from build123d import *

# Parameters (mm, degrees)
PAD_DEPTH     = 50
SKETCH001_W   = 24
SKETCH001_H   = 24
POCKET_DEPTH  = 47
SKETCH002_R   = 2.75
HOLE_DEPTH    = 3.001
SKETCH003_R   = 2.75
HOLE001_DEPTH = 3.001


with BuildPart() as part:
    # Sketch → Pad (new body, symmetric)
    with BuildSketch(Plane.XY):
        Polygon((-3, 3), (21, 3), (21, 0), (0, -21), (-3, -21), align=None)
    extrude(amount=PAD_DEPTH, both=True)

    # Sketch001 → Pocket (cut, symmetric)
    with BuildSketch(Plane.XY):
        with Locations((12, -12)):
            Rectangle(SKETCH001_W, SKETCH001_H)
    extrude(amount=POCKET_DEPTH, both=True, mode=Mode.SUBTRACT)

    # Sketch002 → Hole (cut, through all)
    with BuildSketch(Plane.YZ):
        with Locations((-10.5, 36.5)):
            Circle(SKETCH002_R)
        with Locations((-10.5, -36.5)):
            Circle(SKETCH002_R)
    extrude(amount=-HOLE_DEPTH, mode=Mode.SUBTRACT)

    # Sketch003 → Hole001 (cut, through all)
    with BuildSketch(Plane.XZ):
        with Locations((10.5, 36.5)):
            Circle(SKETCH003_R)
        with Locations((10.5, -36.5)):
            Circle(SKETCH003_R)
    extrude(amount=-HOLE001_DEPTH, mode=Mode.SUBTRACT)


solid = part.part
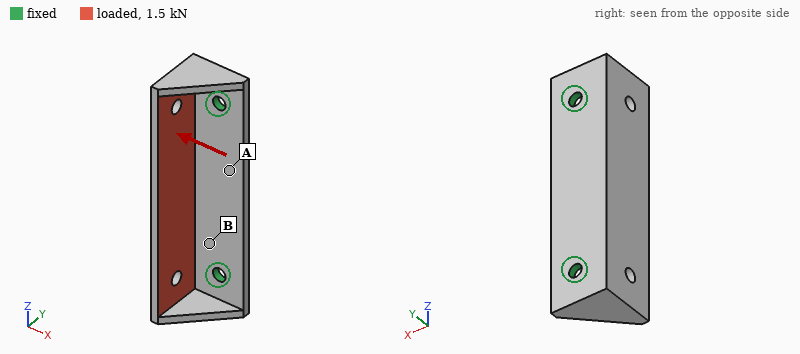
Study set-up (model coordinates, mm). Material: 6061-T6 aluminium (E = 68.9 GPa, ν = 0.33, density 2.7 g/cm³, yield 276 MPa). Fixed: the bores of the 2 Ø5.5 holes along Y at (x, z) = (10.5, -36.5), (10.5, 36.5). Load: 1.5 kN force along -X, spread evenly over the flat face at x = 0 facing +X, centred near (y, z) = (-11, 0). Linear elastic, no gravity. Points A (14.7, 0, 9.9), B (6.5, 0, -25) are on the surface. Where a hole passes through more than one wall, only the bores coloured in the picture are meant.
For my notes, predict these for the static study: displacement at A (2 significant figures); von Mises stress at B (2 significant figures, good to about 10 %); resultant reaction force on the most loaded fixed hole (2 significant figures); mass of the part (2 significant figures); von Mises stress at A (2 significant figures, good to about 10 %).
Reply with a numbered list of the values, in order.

1. 0.11 mm
2. 86 MPa
3. 780 N
4. 39 g
5. 38 MPa
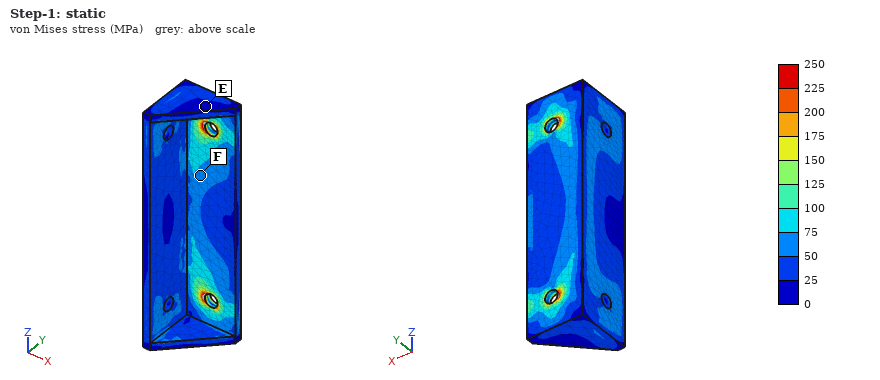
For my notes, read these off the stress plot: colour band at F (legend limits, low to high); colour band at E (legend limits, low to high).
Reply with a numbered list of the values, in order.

1. 50 to 75 MPa
2. 0 to 25 MPa
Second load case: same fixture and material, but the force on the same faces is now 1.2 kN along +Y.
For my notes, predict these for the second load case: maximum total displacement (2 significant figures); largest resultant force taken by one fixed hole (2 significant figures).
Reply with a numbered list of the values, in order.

1. 0.10 mm
2. 620 N
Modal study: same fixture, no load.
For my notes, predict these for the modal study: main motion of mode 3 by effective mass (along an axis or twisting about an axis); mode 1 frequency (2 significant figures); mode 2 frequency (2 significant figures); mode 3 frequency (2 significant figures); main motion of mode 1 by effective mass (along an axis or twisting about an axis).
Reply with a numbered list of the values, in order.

1. along Y
2. 2700 Hz
3. 4000 Hz
4. 4500 Hz
5. along X
